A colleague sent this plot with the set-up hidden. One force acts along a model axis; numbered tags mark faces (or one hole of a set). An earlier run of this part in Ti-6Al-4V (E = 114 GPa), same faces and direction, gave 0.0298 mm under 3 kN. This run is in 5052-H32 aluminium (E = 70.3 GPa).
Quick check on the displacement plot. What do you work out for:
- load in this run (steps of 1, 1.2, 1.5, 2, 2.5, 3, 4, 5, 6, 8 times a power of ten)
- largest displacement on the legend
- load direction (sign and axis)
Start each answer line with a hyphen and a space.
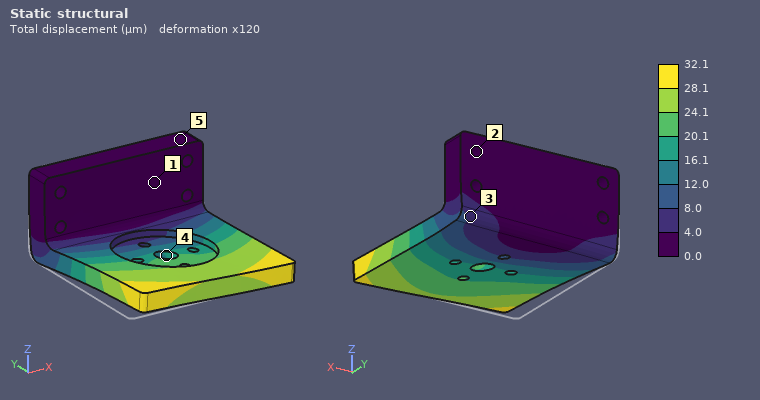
- 2 kN
- 32.1 µm
- +X
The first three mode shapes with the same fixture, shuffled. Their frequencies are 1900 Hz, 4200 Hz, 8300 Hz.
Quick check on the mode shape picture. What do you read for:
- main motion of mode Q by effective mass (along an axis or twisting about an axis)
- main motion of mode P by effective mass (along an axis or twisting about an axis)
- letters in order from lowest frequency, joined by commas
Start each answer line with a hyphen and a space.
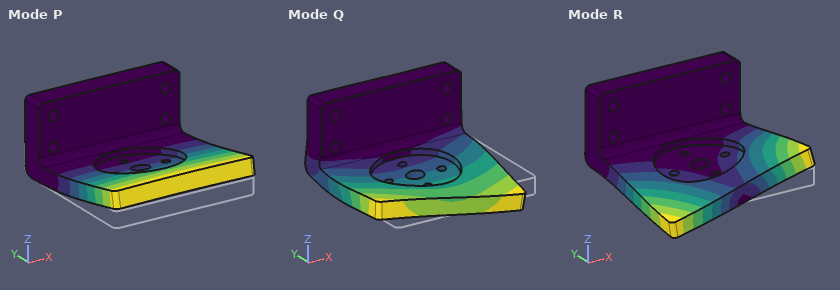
- along X
- along Z
- P, R, Q
